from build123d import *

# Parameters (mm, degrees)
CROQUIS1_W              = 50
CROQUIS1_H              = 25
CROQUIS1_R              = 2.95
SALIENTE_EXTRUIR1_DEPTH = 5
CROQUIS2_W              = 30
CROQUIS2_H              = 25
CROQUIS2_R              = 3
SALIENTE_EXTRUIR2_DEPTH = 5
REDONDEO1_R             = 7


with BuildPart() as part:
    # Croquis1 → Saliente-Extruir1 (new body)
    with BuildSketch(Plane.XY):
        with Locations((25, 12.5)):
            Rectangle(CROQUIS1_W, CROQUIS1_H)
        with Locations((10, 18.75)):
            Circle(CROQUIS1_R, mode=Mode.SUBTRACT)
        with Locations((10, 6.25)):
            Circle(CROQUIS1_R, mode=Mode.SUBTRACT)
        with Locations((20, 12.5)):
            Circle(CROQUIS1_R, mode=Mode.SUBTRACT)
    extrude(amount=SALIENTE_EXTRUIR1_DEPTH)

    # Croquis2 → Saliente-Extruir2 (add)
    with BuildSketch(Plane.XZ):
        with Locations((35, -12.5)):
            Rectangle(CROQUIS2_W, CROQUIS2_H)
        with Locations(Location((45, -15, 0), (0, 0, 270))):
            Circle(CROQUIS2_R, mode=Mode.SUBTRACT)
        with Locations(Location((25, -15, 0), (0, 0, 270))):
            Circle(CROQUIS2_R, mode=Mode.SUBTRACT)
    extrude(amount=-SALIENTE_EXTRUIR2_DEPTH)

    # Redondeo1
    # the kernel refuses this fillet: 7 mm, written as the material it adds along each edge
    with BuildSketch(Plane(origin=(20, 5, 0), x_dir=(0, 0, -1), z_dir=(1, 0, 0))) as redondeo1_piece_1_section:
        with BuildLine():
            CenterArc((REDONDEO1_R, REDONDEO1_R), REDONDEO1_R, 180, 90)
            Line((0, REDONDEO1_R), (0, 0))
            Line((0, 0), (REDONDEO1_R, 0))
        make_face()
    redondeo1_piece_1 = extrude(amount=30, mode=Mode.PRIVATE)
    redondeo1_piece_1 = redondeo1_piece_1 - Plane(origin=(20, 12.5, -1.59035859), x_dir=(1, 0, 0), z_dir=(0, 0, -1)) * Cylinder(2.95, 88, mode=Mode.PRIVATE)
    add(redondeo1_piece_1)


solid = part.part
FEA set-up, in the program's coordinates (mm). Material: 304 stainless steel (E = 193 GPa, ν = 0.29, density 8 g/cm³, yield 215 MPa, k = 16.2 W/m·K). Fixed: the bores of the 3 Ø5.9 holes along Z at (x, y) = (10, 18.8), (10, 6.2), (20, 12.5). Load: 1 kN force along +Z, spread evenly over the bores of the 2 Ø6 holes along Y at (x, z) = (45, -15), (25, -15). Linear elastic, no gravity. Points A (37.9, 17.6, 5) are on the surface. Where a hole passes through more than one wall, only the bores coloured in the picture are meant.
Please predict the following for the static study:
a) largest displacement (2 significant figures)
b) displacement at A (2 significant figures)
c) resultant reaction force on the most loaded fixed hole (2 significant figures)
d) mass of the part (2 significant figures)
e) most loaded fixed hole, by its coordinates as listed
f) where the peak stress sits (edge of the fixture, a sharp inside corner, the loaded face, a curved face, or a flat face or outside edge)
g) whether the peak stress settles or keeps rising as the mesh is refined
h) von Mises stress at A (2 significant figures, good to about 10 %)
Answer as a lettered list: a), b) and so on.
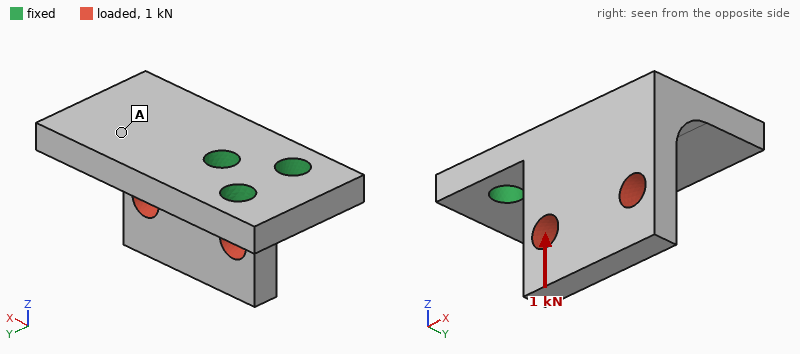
a) 79 µm
b) 16 µm
c) 1.3 kN
d) 77 g
e) (20, 12.5)
f) edge of the fixture
g) keeps rising
h) 24 MPa
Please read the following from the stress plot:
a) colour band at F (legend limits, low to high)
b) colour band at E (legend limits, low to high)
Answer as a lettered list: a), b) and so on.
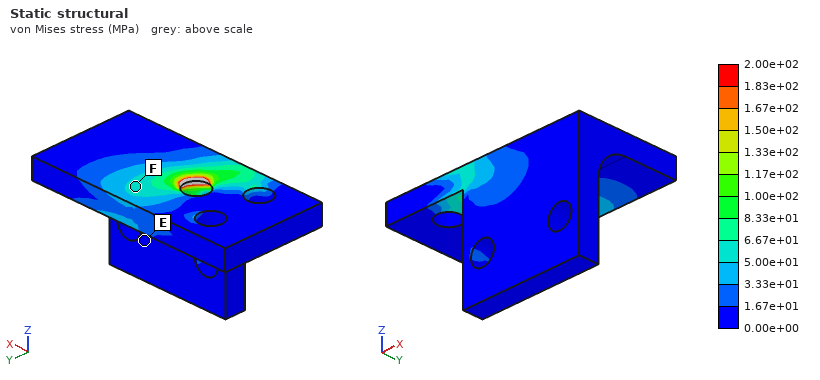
a) 5.00e+01 to 6.67e+01 MPa
b) 0.00e+00 to 1.67e+01 MPa
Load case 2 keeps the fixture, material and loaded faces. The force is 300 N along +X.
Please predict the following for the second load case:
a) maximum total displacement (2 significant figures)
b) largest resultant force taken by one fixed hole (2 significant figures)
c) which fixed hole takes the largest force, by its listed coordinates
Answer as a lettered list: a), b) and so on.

a) 26 µm
b) 290 N
c) (20, 12.5)
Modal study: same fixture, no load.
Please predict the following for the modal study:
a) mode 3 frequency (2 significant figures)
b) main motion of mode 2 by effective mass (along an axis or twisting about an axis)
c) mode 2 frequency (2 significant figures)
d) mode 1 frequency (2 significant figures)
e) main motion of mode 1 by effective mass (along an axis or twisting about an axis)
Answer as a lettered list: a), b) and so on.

a) 9900 Hz
b) along Y
c) 4400 Hz
d) 3000 Hz
e) along Z
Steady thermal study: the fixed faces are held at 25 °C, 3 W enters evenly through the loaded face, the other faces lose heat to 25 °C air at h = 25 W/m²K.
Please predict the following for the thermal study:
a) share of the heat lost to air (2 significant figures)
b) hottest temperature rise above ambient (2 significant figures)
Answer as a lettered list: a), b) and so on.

a) 41 %
b) 28 K
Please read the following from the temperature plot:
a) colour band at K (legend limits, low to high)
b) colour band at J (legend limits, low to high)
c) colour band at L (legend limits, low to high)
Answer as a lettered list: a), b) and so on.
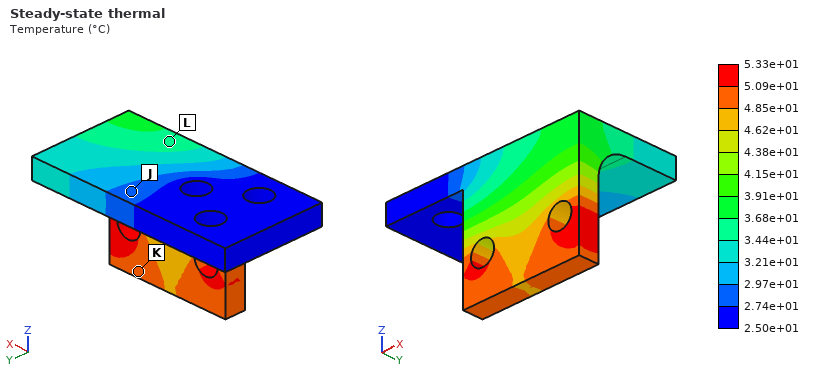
a) 4.85e+01 to 5.09e+01 °C
b) 2.74e+01 to 2.97e+01 °C
c) 3.44e+01 to 3.68e+01 °C
